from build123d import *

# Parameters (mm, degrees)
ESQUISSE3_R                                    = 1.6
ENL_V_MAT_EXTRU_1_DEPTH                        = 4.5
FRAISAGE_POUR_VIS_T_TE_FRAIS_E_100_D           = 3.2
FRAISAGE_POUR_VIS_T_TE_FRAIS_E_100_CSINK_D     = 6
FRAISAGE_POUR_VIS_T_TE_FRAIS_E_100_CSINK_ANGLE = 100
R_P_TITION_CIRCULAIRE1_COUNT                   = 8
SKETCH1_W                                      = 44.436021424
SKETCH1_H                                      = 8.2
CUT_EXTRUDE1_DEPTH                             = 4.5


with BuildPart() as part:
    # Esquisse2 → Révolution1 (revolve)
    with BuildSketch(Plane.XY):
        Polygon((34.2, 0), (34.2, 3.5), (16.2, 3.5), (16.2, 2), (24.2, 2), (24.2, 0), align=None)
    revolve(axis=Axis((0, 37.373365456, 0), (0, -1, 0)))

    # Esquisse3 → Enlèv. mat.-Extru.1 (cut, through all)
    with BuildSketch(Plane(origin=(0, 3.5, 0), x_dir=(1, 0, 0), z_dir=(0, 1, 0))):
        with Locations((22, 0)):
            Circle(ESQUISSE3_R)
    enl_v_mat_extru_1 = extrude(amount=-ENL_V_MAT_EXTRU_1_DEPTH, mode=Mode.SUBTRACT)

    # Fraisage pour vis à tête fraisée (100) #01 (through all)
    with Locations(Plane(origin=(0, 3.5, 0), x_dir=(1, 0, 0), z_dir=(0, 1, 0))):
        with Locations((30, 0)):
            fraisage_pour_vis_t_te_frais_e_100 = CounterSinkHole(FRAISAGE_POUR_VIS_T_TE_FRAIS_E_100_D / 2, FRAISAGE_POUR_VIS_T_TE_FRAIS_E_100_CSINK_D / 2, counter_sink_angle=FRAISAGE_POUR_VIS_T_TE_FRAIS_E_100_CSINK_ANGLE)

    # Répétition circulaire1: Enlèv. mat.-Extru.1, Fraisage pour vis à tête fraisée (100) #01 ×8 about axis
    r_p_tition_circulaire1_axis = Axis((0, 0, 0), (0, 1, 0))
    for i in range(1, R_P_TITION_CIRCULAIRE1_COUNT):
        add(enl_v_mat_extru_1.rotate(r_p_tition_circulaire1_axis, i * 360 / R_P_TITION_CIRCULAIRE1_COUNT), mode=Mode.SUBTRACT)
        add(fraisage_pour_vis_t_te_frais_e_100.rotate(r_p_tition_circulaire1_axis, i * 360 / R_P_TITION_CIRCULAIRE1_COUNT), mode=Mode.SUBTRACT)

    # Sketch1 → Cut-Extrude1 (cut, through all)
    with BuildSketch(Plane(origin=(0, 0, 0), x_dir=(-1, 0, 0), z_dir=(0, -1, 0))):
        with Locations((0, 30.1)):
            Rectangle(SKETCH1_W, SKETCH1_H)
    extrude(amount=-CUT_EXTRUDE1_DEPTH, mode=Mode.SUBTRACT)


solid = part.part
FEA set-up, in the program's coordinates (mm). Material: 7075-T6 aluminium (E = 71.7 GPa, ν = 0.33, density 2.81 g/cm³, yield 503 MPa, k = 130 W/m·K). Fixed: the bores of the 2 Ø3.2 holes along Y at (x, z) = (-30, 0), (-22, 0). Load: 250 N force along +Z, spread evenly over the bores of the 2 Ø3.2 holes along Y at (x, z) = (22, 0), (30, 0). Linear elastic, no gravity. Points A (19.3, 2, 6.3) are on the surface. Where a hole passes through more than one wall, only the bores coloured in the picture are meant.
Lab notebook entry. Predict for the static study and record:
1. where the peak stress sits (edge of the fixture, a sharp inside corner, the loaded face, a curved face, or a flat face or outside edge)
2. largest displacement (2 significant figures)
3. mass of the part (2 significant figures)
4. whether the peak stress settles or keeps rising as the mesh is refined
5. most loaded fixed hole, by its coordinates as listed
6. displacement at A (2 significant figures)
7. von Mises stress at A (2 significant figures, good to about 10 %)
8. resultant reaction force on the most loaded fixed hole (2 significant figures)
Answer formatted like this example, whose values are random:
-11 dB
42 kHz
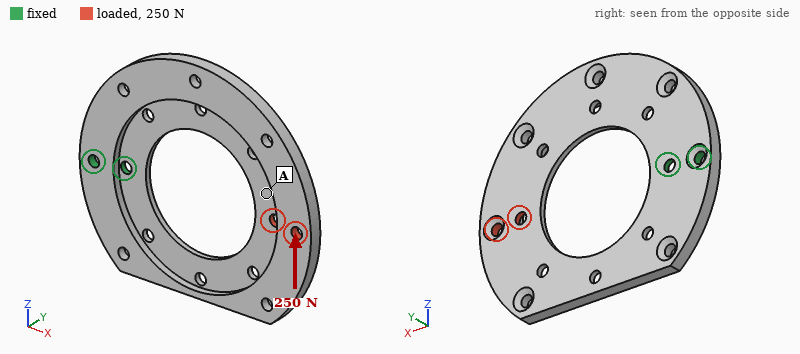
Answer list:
edge of the fixture
0.23 mm
19 g
keeps rising
(-22, 0)
0.13 mm
16 MPa
1.3 kN
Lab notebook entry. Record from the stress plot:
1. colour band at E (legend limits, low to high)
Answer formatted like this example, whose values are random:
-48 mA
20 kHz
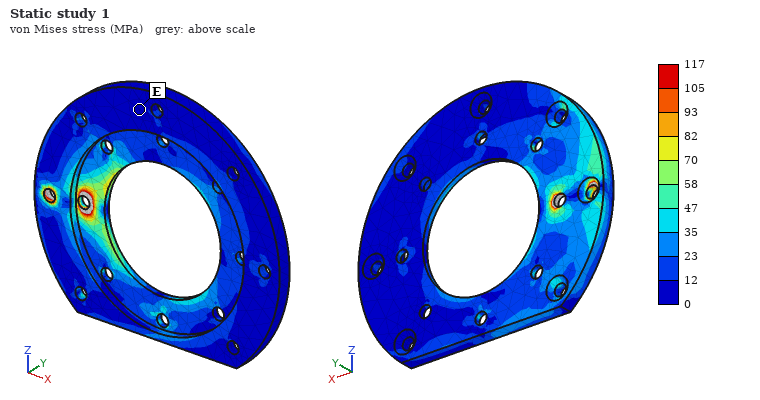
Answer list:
0 to 12 MPa
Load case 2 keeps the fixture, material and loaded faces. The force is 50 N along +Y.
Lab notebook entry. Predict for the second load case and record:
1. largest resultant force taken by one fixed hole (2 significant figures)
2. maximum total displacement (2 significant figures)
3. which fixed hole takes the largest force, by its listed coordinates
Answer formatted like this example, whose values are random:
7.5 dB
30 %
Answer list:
270 N
1.0 mm
(-22, 0)
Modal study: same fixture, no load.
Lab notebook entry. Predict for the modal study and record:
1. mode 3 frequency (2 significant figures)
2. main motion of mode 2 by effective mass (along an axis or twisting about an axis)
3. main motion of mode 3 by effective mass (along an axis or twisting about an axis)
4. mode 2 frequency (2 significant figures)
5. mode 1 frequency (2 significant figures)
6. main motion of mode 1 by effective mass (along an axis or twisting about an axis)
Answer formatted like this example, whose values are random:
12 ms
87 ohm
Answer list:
2300 Hz
twisting about X
along Y
990 Hz
470 Hz
along Y
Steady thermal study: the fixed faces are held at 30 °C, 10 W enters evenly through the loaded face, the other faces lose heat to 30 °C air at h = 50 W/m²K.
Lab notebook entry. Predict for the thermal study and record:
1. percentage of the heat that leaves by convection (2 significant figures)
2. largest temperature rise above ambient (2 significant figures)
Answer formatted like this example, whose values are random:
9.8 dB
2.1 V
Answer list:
62 %
47 K
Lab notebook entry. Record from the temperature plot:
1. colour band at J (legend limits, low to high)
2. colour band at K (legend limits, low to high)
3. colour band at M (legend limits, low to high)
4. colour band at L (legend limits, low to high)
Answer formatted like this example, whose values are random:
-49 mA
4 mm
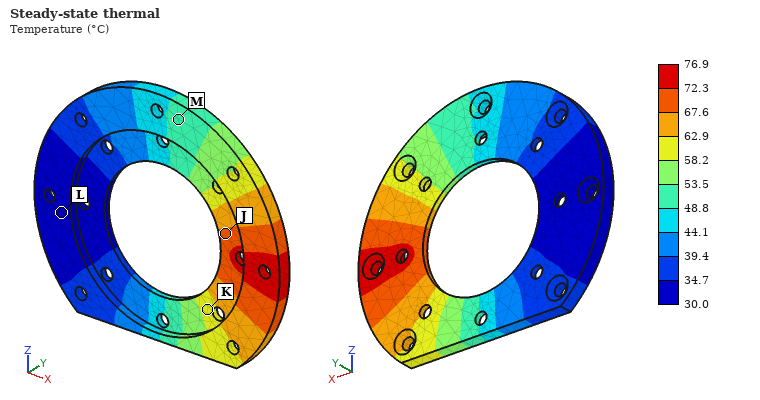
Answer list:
67.6 to 72.3 °C
58.2 to 62.9 °C
48.8 to 53.5 °C
30.0 to 34.7 °C
